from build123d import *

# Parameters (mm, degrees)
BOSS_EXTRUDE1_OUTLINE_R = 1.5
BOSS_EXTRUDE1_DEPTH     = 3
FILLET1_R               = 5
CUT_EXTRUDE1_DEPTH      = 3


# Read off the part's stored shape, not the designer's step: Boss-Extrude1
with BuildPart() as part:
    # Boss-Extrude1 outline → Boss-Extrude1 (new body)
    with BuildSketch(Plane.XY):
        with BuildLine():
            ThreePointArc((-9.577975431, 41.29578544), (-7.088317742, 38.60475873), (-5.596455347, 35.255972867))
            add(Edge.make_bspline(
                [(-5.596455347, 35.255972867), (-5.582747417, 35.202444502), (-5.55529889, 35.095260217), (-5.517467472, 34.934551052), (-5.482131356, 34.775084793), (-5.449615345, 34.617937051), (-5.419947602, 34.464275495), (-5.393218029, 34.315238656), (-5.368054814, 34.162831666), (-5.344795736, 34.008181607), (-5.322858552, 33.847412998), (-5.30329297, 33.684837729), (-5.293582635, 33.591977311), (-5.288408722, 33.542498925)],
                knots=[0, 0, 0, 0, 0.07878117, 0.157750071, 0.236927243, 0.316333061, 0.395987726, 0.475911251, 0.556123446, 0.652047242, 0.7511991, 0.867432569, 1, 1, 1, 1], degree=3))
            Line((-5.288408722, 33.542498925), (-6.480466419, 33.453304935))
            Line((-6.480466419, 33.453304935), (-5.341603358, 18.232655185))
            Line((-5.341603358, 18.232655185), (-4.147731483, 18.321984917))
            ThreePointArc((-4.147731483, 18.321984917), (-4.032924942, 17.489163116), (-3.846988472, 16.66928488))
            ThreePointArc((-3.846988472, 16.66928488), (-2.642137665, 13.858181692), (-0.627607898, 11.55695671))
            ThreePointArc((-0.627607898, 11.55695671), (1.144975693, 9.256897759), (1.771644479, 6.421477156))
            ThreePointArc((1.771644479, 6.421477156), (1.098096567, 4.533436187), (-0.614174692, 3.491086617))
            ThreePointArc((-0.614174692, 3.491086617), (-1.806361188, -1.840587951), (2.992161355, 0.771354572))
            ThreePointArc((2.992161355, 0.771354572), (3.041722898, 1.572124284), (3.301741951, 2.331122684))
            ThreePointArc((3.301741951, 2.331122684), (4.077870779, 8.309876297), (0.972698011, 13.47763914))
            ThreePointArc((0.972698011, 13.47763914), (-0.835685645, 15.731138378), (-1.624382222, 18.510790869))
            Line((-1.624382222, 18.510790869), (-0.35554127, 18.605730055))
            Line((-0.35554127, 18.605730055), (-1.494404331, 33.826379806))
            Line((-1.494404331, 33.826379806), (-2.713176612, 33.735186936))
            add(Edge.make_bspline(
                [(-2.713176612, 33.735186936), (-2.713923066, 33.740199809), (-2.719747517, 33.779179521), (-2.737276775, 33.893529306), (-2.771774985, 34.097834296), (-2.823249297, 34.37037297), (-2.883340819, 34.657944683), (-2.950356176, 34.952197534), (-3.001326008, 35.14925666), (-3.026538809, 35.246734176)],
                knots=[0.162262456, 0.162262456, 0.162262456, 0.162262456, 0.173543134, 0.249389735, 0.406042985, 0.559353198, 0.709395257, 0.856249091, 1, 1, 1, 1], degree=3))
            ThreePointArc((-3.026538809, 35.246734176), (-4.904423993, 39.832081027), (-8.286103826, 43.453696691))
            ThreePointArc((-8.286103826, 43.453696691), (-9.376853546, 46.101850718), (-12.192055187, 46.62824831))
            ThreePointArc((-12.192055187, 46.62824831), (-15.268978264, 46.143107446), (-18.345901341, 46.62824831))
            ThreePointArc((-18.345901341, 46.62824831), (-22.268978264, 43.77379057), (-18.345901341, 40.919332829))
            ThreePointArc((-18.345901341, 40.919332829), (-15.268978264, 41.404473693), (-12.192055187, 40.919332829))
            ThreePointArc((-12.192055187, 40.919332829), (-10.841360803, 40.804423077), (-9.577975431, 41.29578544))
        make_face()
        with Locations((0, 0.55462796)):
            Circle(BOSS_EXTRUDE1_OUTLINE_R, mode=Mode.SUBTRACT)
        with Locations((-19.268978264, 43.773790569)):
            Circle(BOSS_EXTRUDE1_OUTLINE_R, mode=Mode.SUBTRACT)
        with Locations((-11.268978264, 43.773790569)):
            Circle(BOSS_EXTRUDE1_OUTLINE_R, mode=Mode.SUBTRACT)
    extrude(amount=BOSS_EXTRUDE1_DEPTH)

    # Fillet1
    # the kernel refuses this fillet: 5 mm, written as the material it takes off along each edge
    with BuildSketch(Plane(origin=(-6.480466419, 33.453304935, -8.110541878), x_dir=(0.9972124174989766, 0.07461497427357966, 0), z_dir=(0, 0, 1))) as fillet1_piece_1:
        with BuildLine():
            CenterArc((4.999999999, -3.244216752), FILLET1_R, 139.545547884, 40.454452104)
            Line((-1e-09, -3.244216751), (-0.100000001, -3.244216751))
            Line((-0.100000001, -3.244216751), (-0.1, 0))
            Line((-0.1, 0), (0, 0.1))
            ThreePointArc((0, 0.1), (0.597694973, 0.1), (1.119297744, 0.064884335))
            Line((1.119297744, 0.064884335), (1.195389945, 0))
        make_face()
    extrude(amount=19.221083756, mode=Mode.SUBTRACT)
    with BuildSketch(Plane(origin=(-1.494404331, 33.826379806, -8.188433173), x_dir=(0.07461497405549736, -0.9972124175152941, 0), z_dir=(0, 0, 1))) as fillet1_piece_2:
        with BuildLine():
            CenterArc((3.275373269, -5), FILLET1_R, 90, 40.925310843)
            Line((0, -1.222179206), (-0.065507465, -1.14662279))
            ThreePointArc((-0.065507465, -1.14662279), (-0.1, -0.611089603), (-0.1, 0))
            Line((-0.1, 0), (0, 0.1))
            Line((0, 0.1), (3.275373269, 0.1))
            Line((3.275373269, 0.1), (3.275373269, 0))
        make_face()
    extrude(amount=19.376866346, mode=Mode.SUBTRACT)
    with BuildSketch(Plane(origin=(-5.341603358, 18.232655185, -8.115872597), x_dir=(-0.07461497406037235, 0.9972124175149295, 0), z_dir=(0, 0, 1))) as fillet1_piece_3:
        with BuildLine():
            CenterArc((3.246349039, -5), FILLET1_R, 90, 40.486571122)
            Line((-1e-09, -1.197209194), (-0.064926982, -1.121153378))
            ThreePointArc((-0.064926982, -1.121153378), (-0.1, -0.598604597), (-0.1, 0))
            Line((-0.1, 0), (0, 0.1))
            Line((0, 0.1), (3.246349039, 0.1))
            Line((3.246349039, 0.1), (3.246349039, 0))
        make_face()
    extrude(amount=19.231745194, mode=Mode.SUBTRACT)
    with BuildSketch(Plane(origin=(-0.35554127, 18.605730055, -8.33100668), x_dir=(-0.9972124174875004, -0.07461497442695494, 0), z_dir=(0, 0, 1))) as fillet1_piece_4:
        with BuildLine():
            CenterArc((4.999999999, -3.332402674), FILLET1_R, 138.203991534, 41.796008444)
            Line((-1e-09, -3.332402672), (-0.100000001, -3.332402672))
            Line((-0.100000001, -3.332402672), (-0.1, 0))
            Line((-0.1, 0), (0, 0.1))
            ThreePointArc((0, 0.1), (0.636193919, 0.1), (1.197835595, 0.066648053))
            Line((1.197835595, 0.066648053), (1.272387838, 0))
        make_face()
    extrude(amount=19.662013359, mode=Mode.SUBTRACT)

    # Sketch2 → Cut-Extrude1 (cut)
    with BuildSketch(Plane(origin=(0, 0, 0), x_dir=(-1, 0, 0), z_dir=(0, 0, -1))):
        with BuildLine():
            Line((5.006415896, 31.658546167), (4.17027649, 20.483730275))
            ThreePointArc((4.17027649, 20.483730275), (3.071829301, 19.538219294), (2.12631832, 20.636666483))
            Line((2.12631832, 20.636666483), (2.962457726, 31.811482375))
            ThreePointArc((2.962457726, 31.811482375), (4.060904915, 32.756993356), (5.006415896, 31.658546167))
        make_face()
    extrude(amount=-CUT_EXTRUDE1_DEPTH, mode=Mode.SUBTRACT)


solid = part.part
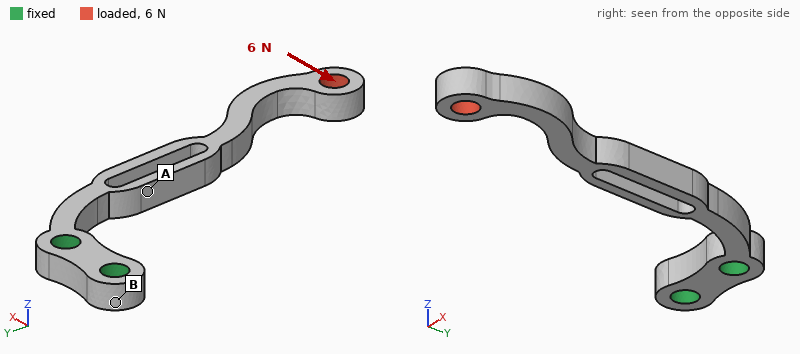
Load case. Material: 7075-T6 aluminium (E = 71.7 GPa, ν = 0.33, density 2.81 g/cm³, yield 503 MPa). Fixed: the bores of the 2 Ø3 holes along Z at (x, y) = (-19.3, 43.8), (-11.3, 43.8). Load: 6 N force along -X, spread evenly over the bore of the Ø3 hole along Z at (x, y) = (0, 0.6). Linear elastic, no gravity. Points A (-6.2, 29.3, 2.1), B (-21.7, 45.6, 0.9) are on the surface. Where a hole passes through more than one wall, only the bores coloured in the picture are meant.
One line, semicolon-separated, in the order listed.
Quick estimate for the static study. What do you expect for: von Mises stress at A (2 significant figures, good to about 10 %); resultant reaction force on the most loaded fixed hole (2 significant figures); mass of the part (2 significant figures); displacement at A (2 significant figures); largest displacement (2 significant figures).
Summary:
16 MPa; 5.8 N; 1.6 g; 0.097 mm; 0.53 mm
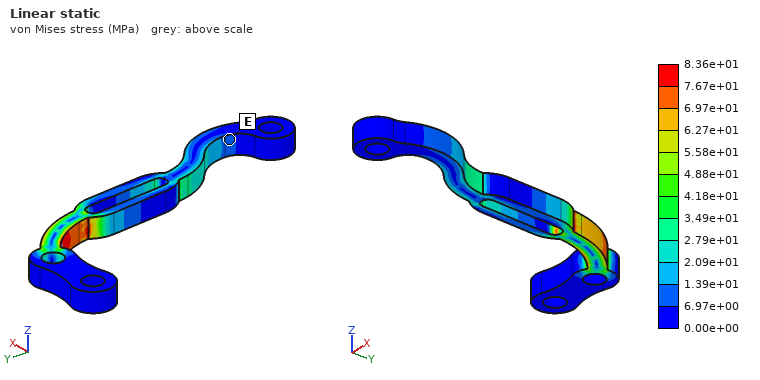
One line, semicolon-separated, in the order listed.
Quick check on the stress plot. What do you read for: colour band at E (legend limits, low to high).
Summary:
6.97e+00 to 1.39e+01 MPa
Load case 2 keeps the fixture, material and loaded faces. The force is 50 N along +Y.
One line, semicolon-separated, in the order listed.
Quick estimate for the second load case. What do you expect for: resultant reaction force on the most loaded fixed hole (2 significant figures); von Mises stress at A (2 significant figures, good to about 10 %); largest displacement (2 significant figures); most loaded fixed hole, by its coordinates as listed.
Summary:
60 N; 13 MPa; 0.61 mm; (-11.3, 43.8)
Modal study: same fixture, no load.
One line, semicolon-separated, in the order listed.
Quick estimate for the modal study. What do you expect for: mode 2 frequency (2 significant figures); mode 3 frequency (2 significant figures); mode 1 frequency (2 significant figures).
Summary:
880 Hz; 5500 Hz; 860 Hz
